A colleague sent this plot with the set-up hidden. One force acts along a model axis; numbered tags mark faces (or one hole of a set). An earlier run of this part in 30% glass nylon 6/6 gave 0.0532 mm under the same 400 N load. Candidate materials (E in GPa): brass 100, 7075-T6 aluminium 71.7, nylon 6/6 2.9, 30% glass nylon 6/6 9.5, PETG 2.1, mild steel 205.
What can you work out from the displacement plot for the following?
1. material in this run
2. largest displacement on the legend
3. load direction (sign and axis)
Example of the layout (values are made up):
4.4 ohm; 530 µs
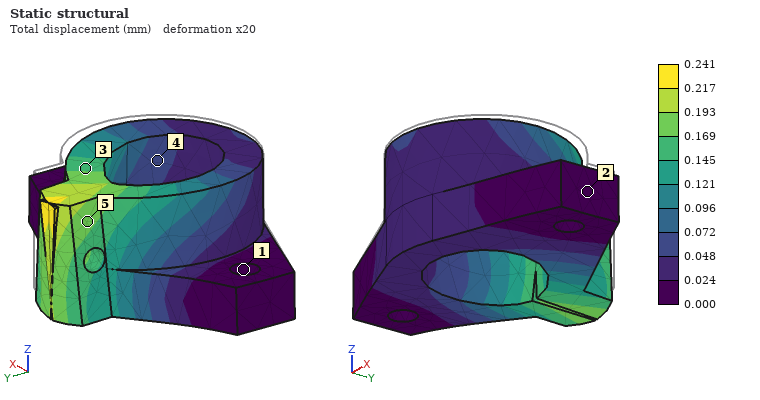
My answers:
PETG; 0.241 mm; -Z
